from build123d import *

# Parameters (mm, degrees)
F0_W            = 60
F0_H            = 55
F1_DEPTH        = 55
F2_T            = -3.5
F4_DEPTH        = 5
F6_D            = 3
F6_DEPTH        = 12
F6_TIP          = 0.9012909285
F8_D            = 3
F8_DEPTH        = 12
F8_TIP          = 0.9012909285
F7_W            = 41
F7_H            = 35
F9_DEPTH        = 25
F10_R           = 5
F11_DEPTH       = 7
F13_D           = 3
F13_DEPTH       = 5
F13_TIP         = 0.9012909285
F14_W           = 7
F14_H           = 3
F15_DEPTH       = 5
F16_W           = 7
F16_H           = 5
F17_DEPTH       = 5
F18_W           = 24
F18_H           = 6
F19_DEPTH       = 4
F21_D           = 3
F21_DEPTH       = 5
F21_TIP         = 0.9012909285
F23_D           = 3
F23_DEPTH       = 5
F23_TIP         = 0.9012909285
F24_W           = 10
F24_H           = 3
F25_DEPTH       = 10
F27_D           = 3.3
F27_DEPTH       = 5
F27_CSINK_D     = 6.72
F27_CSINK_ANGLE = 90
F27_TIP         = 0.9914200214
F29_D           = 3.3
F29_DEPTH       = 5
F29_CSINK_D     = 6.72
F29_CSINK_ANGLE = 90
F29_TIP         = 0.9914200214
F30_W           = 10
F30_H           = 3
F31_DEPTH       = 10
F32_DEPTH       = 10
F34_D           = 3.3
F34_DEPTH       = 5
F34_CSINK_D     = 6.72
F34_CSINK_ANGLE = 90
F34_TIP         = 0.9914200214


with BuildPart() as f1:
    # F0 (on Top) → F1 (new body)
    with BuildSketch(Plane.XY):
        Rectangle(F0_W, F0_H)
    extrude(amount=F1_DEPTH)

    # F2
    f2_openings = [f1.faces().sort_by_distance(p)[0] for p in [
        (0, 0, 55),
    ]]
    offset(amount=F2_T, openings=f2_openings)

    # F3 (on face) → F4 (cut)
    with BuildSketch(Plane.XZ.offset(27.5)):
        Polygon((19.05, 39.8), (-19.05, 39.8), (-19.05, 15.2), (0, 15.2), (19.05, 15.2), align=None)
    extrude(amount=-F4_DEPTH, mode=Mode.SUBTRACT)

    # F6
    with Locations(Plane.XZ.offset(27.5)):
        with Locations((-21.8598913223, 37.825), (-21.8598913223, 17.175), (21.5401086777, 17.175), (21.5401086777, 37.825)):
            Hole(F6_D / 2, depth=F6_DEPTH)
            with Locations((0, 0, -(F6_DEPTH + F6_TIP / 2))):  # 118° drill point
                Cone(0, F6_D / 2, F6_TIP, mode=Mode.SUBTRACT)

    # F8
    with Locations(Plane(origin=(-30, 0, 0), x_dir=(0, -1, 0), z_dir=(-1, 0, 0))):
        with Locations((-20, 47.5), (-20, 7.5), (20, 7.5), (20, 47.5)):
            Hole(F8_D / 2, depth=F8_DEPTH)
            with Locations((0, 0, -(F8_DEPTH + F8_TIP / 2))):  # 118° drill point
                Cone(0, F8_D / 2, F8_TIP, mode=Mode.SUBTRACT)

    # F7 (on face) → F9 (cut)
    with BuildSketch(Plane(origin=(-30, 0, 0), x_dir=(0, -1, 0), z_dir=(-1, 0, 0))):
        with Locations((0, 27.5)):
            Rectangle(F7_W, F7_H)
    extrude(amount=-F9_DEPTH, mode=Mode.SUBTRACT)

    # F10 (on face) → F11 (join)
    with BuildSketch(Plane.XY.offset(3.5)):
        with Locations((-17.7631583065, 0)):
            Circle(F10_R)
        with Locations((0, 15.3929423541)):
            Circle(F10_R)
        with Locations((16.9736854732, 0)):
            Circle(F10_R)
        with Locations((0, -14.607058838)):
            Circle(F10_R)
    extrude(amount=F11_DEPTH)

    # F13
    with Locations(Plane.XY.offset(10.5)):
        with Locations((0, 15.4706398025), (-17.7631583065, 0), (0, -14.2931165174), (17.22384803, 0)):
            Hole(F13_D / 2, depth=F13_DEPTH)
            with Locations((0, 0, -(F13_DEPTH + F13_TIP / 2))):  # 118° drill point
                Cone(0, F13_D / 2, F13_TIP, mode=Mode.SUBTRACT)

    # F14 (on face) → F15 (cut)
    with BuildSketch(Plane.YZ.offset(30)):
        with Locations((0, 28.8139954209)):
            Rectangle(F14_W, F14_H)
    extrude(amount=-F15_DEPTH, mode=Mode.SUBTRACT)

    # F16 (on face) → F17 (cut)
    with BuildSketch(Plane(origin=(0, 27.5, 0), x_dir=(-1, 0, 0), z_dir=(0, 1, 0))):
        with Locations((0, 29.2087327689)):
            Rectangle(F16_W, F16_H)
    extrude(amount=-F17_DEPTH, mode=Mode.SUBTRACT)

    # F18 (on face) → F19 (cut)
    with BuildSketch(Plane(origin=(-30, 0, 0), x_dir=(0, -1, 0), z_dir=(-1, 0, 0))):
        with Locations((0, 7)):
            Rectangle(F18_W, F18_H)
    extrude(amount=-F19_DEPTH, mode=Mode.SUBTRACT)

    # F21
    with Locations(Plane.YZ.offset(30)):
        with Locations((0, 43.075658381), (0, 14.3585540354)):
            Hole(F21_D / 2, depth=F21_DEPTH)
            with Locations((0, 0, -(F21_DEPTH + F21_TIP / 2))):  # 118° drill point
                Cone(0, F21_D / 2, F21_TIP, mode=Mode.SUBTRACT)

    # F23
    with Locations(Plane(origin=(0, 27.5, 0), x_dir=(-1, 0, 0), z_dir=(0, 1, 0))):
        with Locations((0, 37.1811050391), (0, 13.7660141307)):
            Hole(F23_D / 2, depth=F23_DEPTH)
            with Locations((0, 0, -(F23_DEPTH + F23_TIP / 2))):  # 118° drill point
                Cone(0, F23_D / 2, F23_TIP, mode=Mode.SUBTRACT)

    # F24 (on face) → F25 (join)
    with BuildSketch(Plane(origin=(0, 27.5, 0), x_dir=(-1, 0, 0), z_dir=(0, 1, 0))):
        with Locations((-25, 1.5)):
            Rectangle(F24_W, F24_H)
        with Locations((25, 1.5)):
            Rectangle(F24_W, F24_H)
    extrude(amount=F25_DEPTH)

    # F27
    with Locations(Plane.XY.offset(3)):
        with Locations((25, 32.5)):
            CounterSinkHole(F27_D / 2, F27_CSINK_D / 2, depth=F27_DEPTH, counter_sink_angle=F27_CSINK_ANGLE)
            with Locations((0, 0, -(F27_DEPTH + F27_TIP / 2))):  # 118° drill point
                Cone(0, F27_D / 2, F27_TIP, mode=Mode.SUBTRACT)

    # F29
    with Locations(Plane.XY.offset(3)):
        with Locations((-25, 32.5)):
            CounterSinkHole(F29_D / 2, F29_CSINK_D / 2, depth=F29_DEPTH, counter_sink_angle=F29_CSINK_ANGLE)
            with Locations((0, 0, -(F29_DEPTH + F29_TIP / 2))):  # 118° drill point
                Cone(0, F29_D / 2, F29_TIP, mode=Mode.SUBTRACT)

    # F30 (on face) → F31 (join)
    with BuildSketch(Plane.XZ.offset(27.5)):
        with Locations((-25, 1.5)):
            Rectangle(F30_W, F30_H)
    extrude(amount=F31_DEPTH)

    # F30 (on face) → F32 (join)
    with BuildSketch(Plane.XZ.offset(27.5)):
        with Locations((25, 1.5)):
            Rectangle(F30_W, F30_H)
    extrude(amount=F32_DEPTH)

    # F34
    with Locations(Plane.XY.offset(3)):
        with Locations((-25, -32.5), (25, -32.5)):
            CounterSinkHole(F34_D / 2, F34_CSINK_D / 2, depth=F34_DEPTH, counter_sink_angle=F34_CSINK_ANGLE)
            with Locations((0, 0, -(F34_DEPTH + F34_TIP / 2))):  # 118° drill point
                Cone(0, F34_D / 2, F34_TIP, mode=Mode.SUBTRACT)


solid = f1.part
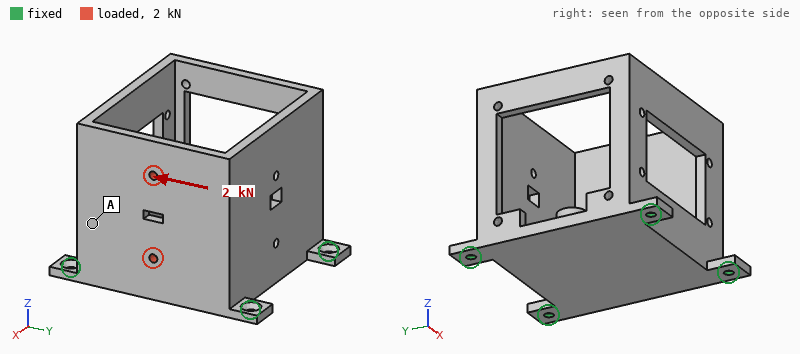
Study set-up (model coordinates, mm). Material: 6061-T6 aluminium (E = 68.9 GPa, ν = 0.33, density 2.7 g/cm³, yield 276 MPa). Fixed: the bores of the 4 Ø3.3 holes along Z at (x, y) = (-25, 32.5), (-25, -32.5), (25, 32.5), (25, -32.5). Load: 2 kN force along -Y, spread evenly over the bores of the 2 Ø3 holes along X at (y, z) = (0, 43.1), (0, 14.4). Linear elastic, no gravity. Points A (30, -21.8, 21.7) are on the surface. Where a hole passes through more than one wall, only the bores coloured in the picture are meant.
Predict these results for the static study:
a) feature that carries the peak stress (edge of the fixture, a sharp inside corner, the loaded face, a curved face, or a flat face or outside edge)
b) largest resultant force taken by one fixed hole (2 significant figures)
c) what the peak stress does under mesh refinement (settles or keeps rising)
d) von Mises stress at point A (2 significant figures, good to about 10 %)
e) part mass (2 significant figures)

edge of the fixture
1.3 kN
keeps rising
9.6 MPa
120 g
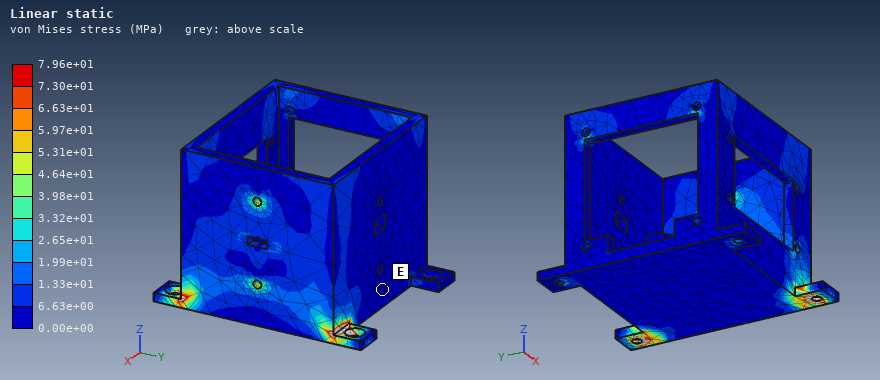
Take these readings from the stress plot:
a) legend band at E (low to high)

0.00e+00 to 6.63e+00 MPa
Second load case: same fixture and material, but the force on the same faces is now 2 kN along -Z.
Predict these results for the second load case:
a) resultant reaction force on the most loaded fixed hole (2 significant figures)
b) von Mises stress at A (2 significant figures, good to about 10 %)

1.4 kN
13 MPa
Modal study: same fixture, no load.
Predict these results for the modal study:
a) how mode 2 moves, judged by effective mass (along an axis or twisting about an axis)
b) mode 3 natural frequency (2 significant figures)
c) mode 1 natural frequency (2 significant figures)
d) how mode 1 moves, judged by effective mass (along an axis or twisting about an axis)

along X
3300 Hz
2000 Hz
along Y
